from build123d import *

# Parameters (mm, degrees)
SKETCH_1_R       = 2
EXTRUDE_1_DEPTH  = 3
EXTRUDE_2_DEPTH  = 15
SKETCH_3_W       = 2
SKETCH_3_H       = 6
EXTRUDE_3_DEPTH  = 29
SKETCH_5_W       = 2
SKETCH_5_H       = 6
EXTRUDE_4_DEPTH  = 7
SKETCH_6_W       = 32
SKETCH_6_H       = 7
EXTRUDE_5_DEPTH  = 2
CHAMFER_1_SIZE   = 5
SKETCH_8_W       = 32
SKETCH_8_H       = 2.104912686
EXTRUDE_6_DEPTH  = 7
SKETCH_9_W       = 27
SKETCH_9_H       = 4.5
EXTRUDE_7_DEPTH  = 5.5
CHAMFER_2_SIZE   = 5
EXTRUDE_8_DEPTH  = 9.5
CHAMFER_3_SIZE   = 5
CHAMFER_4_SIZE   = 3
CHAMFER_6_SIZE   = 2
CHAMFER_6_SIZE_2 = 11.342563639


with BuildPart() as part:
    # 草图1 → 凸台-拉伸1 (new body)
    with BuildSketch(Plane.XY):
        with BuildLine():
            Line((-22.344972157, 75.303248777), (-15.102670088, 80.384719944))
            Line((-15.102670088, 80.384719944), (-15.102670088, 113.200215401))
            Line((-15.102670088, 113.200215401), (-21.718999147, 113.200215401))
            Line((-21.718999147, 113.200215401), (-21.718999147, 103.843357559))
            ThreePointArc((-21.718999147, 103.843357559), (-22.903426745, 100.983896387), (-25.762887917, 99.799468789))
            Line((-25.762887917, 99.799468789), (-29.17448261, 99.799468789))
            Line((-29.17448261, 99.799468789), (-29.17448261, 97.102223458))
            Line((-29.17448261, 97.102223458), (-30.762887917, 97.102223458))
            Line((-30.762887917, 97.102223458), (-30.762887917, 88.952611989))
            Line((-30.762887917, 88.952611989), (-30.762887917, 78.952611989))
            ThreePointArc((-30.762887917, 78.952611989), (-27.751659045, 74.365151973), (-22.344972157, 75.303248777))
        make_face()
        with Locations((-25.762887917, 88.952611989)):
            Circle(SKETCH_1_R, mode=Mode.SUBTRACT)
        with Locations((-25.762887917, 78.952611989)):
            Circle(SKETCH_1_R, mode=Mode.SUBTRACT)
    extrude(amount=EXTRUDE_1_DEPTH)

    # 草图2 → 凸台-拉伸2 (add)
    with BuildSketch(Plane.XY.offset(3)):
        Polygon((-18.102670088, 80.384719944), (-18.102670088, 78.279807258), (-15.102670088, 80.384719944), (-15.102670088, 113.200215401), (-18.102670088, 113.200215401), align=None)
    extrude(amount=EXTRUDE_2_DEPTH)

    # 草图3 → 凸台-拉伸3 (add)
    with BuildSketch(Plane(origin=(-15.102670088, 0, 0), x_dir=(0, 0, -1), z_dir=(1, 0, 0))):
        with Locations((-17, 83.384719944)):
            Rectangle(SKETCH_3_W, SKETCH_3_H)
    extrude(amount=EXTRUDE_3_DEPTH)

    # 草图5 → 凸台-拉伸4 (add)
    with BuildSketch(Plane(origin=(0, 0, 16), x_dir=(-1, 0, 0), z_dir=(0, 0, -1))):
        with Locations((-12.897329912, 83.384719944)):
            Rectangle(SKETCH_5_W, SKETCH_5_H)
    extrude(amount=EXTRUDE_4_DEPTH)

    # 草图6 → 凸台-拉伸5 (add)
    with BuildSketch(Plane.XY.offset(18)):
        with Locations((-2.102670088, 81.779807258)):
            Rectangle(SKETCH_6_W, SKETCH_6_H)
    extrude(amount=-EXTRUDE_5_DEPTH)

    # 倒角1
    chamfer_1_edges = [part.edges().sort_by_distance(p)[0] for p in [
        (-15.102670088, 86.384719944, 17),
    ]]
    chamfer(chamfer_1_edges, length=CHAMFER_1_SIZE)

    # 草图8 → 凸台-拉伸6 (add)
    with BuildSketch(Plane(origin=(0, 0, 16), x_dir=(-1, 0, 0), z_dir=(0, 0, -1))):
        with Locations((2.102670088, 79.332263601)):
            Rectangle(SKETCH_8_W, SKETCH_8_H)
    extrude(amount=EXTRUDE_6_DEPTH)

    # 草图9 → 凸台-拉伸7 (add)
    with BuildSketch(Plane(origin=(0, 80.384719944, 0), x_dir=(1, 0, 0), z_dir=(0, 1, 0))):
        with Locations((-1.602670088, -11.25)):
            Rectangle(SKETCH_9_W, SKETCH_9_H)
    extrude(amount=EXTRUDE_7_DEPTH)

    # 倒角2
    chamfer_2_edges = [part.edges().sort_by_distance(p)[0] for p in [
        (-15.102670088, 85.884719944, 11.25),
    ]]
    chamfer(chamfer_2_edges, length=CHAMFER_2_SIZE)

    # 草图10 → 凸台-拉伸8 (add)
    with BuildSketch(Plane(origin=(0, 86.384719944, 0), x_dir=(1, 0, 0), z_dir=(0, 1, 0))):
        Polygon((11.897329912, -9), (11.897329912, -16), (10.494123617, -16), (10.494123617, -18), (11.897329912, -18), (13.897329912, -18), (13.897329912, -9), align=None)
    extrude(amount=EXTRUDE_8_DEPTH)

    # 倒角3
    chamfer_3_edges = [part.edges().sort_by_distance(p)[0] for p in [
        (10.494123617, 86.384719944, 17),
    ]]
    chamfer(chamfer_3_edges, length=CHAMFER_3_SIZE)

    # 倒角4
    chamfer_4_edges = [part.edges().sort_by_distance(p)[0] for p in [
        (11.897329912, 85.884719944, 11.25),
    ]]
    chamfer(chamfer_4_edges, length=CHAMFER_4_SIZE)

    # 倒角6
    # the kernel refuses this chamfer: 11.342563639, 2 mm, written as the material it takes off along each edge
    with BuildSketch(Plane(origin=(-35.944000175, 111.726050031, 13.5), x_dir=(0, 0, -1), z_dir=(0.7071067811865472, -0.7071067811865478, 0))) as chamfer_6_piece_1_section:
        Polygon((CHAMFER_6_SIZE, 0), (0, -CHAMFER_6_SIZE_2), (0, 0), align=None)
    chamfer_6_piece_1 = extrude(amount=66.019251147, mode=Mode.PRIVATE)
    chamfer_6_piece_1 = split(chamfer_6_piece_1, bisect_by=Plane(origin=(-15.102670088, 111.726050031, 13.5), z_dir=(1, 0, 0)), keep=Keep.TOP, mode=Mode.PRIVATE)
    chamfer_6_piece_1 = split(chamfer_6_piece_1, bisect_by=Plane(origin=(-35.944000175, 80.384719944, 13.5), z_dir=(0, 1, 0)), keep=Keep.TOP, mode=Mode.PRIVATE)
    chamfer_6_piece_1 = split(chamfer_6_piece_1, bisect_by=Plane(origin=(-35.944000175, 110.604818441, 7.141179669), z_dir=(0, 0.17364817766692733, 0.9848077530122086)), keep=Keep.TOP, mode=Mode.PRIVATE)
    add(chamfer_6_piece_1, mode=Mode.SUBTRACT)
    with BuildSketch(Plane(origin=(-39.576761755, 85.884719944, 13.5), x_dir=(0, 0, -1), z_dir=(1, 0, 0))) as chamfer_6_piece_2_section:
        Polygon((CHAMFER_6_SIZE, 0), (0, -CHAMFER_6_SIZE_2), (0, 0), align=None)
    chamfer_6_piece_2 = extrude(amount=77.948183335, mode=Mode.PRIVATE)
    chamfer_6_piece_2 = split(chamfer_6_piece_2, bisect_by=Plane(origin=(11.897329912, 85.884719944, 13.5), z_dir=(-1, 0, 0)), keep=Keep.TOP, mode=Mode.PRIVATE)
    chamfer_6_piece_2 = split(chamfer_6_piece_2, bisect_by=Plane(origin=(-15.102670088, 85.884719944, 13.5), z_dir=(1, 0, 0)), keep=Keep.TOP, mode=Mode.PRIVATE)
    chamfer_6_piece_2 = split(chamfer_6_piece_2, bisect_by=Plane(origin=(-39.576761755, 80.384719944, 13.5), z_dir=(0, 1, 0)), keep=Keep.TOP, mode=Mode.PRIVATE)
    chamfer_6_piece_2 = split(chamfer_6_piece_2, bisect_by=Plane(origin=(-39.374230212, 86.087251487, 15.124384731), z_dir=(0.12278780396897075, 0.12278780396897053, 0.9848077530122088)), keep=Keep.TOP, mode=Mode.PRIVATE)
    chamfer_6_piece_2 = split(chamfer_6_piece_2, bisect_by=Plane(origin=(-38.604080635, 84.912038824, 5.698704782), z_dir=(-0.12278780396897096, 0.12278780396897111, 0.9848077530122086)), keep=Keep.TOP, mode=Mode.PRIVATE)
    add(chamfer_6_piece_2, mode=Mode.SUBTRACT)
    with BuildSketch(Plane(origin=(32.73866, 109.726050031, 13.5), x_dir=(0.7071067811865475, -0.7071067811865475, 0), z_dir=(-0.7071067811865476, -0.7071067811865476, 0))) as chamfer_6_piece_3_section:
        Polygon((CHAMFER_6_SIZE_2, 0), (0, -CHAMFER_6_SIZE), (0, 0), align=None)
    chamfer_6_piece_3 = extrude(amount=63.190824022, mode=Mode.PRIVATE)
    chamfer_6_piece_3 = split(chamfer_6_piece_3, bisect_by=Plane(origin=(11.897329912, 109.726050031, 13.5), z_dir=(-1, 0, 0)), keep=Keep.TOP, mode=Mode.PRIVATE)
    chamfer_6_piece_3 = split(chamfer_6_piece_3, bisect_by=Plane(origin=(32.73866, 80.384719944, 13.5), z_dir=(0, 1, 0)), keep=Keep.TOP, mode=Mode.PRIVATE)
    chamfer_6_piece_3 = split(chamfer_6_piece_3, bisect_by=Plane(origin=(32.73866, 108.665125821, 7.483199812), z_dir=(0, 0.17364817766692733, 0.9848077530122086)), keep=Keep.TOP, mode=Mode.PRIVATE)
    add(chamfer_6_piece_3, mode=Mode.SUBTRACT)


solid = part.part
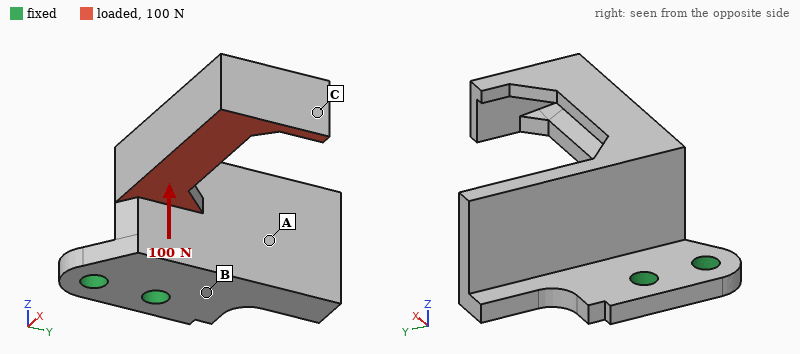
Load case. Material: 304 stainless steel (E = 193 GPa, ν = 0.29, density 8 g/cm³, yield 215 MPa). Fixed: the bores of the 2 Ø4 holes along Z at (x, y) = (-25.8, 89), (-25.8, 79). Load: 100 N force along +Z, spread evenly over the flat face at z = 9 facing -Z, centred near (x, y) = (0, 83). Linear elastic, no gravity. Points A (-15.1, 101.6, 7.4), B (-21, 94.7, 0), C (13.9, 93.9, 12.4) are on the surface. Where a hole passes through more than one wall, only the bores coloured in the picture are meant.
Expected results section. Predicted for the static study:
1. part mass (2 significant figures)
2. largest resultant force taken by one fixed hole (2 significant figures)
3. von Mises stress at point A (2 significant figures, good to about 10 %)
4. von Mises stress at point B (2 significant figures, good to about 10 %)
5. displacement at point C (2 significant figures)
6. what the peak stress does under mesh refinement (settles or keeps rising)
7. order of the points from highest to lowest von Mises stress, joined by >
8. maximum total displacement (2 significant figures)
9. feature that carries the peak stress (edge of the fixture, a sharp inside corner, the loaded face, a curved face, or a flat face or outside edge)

37 g
51 N
18 MPa
43 MPa
0.13 mm
keeps rising
B > A > C
0.13 mm
edge of the fixture
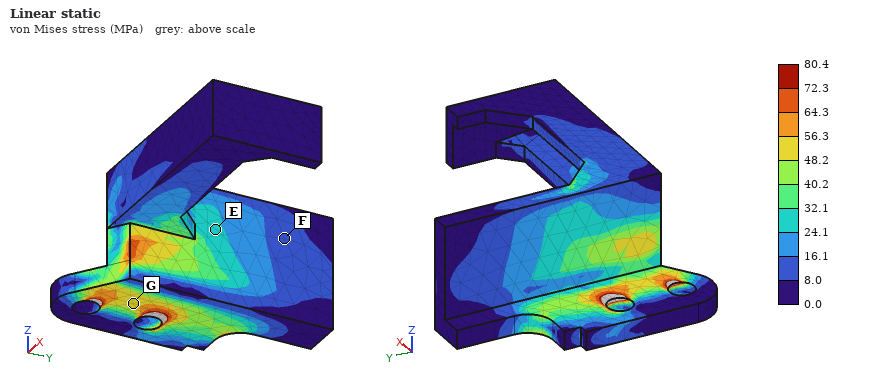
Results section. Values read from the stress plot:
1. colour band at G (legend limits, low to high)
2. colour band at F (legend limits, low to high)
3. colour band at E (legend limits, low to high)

48.2 to 56.3 MPa
8.0 to 16.1 MPa
24.1 to 32.1 MPa
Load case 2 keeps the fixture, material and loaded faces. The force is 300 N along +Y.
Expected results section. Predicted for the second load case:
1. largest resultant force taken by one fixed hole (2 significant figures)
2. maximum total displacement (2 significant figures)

620 N
0.11 mm
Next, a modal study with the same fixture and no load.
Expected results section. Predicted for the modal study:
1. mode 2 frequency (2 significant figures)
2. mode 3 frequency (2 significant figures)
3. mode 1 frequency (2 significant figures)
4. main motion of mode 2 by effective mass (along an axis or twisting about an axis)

2500 Hz
3900 Hz
1200 Hz
along Y
